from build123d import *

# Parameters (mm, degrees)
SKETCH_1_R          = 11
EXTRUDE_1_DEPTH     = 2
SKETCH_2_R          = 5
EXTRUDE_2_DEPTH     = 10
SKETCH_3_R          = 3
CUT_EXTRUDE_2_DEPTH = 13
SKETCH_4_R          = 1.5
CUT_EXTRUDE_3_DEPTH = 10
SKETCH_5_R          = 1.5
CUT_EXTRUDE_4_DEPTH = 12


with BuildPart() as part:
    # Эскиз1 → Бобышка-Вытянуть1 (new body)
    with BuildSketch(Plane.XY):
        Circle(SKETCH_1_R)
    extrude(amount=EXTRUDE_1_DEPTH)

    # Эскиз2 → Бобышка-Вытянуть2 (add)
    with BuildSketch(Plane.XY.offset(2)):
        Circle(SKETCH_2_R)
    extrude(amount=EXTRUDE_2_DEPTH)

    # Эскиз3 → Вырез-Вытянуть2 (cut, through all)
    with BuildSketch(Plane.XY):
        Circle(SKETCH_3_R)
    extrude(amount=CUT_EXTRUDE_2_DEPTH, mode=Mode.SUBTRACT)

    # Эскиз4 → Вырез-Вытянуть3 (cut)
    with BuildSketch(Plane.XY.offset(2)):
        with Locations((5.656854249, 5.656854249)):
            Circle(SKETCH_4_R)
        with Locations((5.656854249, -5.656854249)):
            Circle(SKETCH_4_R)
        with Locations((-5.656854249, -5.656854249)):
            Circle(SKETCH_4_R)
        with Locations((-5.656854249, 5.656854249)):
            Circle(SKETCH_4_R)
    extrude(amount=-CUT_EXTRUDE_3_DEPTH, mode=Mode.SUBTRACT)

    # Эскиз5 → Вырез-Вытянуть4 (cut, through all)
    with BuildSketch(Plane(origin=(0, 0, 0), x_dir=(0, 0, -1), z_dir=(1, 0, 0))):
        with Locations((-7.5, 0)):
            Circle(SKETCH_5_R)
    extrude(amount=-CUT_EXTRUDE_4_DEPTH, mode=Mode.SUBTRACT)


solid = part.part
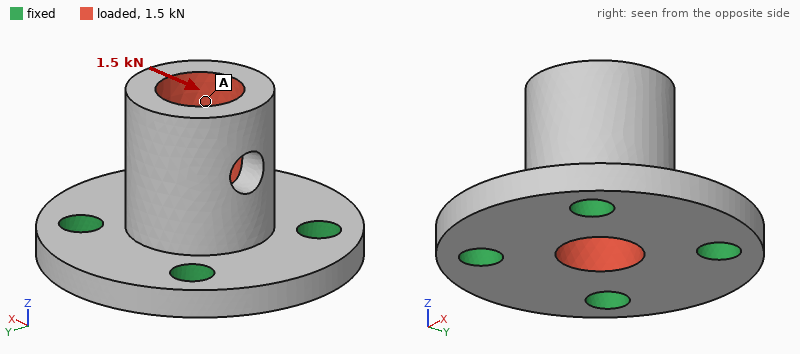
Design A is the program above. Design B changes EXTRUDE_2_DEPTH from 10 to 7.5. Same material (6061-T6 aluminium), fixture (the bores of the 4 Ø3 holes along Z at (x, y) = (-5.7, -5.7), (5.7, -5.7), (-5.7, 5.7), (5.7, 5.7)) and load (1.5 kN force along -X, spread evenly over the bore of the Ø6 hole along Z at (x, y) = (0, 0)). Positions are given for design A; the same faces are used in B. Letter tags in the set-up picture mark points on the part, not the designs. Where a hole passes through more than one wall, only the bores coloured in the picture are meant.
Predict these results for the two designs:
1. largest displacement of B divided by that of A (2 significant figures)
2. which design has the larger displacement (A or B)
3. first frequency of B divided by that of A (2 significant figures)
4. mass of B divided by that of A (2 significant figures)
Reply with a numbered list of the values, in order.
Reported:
1. 0.61
2. A
3. 1.4
4. 0.89
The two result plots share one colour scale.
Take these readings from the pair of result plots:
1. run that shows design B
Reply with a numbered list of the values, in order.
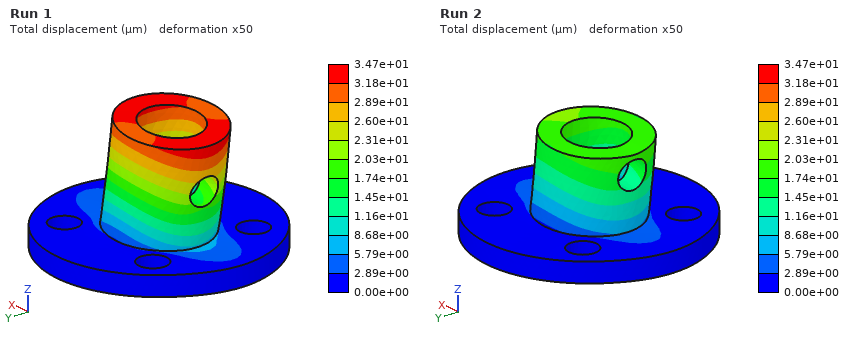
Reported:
1. Run 2
